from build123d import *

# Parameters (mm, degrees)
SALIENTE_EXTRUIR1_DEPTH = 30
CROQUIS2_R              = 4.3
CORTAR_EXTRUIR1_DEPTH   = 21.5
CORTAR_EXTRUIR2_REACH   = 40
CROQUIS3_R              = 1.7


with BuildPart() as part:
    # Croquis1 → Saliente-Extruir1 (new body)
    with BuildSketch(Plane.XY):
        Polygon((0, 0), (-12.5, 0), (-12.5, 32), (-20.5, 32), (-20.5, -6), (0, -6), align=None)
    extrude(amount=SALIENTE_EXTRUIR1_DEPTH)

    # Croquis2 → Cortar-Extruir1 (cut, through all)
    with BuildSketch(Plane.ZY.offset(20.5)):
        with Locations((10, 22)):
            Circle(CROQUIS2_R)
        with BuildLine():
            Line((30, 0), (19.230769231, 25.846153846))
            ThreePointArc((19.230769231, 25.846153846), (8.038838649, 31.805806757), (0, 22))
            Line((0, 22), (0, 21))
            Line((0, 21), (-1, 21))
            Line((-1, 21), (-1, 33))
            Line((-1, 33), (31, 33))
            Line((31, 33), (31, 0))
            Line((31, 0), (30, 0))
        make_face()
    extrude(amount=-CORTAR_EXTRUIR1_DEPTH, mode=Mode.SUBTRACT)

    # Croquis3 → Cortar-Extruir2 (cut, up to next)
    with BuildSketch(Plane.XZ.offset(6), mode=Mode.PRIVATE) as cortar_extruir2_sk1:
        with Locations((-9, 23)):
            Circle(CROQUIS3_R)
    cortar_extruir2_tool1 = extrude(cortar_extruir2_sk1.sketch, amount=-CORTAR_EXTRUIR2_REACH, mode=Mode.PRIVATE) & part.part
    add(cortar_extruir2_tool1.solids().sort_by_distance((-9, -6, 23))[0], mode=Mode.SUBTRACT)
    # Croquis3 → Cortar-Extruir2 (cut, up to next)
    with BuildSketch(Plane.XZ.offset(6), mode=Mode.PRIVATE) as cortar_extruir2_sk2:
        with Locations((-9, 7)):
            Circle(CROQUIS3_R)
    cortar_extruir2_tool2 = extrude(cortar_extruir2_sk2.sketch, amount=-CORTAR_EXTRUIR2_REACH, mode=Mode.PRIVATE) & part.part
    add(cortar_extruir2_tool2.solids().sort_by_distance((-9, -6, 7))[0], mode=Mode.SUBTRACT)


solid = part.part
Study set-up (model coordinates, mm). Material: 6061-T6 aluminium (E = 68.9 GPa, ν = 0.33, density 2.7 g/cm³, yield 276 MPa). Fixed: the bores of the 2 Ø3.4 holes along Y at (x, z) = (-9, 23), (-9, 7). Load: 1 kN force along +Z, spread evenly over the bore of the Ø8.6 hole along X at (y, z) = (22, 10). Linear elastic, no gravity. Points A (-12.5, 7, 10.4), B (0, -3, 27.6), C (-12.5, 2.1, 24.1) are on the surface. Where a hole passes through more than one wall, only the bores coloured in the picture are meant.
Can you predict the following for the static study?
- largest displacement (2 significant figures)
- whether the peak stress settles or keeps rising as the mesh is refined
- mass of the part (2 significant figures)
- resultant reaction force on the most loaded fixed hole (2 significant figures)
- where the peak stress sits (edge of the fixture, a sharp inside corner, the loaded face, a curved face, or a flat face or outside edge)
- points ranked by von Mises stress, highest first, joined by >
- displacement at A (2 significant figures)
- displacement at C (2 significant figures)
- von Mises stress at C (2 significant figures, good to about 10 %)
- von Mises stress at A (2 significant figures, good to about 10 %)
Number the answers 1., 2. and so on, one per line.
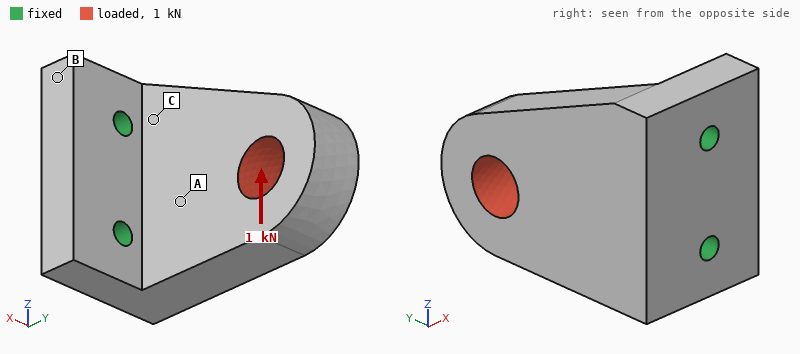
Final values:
1. 46 µm
2. keeps rising
3. 24 g
4. 1.4 kN
5. edge of the fixture
6. C > A > B
7. 13 µm
8. 9.0 µm
9. 41 MPa
10. 20 MPa
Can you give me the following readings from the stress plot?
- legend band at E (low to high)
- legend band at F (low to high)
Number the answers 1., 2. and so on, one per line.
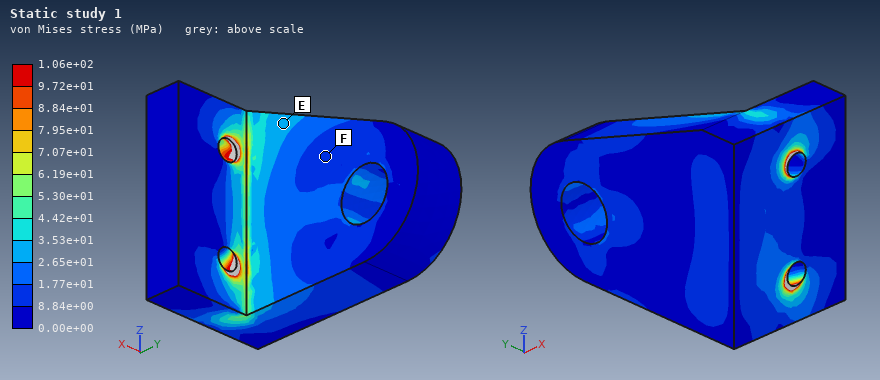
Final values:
1. 2.65e+01 to 3.53e+01 MPa
2. 8.84e+00 to 1.77e+01 MPa
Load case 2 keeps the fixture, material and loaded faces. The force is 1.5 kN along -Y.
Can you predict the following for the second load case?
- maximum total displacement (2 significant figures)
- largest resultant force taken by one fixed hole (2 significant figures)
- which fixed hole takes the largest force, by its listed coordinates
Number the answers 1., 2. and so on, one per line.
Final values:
1. 54 µm
2. 1.1 kN
3. (-9, 7)
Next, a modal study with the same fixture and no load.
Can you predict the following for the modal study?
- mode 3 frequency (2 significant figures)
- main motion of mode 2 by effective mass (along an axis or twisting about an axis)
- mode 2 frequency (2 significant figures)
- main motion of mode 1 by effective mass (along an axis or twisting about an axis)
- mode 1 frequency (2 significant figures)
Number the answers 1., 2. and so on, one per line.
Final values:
1. 17 kHz
2. along Z
3. 9600 Hz
4. along X
5. 4400 Hz
